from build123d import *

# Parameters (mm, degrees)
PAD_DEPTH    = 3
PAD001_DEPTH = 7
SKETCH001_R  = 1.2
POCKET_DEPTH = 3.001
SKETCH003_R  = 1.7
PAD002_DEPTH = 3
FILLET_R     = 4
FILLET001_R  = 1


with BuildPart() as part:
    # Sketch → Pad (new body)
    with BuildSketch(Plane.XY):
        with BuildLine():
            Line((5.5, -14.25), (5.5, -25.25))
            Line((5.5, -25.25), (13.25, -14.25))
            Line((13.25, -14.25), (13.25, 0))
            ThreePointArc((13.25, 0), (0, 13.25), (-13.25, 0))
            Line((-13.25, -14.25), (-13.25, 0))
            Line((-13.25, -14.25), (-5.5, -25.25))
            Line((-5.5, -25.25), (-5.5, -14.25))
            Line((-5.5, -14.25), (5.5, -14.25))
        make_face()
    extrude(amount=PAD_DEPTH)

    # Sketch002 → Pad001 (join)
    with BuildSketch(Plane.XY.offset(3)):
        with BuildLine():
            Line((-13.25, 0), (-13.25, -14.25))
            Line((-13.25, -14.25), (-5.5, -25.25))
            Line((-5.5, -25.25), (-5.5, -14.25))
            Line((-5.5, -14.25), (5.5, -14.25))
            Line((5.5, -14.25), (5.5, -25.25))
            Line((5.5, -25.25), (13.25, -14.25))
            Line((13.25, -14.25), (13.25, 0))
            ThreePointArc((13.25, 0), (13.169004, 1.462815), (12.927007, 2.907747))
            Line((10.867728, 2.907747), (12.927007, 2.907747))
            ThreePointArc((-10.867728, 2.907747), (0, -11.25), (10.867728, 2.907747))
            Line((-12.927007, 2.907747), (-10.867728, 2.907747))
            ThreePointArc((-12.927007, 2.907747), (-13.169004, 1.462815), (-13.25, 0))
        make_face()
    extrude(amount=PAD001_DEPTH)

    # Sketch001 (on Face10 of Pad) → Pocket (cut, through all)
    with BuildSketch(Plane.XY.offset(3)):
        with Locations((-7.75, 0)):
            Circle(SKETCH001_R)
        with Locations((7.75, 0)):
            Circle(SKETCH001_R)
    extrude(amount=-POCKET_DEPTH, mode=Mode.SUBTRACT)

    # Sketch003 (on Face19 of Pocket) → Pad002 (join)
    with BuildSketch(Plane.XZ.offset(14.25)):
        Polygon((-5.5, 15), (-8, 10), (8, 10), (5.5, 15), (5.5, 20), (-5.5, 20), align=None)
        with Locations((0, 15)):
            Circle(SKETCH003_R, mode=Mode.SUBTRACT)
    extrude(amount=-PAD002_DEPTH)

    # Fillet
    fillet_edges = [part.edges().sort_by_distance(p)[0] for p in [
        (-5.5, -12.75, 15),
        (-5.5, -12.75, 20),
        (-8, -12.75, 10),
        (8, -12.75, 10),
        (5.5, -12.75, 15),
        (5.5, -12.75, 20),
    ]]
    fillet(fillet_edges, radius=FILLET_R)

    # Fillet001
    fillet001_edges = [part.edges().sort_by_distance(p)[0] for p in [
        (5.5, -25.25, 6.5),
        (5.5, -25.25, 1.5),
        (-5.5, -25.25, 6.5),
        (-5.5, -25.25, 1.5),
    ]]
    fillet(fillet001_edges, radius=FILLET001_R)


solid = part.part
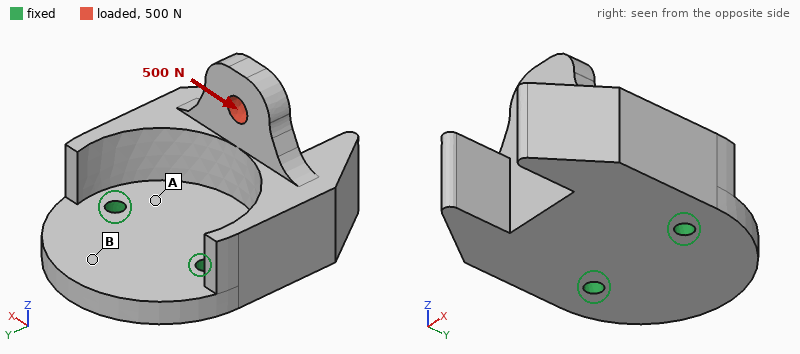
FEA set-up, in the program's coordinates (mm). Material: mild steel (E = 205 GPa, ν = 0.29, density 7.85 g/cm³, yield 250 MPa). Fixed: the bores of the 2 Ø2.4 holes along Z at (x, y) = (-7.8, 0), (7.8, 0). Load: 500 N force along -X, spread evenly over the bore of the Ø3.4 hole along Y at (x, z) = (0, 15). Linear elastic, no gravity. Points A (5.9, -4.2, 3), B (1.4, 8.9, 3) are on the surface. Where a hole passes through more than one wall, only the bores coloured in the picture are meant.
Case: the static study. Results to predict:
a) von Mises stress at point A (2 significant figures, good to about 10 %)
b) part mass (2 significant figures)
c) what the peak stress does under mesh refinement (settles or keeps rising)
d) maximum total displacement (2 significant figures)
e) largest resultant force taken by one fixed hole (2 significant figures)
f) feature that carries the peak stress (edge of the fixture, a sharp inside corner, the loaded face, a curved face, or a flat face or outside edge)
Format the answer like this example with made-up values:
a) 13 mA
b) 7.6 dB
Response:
a) 48 MPa
b) 35 g
c) keeps rising
d) 19 µm
e) 550 N
f) edge of the fixture
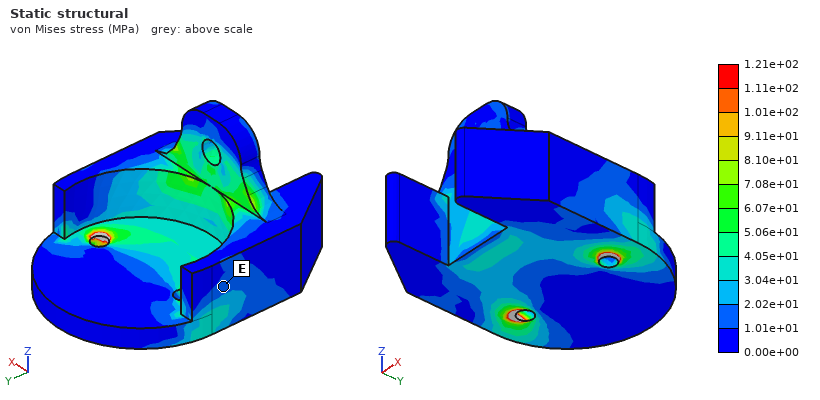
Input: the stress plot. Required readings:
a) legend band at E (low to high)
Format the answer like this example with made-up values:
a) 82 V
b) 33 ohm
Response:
a) 1.01e+01 to 2.02e+01 MPa
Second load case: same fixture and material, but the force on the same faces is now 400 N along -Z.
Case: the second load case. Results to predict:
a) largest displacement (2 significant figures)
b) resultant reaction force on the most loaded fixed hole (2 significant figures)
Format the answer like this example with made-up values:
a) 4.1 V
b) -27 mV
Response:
a) 29 µm
b) 200 N
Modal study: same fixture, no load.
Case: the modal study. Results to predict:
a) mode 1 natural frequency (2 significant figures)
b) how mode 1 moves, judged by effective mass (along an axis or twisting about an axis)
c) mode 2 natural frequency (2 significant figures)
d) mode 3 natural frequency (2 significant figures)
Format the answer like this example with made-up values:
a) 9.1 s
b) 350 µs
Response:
a) 4600 Hz
b) along Z
c) 8600 Hz
d) 17 kHz
